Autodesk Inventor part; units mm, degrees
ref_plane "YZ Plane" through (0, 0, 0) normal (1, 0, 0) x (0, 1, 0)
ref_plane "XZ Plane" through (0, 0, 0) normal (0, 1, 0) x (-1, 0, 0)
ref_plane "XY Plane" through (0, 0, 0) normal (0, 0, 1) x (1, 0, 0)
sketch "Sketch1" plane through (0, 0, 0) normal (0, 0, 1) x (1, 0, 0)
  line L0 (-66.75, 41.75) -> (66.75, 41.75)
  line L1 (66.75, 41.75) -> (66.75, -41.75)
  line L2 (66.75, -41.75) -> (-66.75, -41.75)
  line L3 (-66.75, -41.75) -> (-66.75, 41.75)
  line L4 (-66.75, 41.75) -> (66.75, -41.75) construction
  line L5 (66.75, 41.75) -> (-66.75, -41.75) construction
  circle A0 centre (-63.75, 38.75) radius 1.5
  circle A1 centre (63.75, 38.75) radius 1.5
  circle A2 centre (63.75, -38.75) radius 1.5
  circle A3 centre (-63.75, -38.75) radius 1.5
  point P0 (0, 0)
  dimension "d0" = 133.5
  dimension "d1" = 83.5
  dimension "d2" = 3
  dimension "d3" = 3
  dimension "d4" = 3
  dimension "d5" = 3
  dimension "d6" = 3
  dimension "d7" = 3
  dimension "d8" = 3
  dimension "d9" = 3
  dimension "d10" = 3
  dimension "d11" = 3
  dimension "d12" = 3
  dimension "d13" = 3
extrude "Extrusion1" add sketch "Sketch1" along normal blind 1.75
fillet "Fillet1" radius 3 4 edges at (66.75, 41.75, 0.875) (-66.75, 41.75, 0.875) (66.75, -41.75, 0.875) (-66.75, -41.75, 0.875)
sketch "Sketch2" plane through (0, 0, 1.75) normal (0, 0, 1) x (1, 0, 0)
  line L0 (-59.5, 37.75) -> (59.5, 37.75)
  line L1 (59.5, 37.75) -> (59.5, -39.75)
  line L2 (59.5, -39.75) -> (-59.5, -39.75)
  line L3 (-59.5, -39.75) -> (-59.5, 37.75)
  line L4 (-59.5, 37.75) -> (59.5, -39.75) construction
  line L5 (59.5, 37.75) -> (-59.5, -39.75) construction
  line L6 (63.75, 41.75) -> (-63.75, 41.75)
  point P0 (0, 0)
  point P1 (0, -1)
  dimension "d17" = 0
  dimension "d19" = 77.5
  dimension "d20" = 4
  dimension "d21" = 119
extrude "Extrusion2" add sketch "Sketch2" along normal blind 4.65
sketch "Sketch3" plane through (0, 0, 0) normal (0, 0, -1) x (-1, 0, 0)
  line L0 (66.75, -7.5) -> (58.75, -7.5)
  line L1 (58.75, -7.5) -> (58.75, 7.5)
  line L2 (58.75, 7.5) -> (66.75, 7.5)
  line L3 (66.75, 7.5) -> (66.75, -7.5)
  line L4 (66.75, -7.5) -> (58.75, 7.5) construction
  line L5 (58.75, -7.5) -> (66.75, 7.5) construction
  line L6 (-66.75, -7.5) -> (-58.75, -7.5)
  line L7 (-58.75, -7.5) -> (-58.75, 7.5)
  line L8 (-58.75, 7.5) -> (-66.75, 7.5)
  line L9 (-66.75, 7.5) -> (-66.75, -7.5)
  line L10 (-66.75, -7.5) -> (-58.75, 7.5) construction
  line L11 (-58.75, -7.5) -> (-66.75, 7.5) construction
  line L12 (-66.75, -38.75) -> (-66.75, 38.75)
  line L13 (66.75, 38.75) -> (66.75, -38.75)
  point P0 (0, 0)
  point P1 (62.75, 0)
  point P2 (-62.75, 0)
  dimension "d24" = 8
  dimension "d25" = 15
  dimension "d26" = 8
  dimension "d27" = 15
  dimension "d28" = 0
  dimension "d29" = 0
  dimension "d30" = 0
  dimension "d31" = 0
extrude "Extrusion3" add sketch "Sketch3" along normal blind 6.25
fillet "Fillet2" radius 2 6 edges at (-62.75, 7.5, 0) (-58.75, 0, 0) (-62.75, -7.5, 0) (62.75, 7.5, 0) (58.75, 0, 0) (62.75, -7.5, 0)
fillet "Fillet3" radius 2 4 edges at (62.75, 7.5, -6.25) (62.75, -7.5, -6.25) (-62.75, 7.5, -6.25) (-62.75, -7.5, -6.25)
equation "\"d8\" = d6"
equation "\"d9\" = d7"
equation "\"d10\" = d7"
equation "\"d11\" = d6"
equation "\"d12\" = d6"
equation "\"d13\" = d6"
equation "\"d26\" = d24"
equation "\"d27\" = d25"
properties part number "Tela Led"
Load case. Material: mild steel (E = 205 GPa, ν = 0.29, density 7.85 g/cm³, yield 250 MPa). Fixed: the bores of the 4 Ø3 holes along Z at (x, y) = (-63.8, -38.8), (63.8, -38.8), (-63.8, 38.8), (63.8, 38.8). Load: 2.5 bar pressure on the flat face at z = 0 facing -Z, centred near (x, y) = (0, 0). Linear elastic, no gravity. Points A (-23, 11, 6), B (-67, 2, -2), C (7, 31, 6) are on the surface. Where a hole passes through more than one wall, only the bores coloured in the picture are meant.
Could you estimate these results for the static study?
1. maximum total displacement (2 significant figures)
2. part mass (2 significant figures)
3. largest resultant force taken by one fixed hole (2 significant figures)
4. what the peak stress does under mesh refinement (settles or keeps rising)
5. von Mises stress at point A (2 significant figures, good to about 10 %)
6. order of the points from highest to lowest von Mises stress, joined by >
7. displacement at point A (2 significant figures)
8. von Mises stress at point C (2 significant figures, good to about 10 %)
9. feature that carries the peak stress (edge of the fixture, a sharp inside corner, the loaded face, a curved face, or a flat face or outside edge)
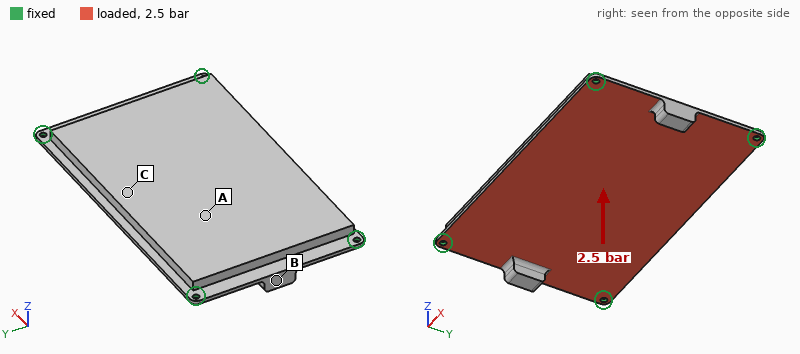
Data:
0.15 mm
500 g
2.1 kN
keeps rising
44 MPa
C > A > B
0.12 mm
63 MPa
edge of the fixture
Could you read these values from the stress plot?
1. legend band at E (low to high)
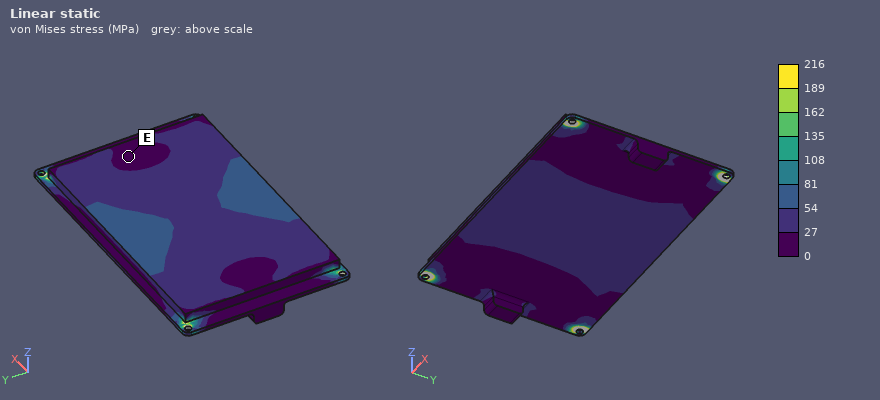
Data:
0 to 27 MPa
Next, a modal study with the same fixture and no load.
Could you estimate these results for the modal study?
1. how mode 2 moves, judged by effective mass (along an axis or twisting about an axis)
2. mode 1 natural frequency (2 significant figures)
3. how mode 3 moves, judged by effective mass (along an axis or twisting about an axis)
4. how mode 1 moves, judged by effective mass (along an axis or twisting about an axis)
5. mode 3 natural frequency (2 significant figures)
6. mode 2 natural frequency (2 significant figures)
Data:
twisting about X
1100 Hz
twisting about Y
along Z
2600 Hz
2200 Hz
